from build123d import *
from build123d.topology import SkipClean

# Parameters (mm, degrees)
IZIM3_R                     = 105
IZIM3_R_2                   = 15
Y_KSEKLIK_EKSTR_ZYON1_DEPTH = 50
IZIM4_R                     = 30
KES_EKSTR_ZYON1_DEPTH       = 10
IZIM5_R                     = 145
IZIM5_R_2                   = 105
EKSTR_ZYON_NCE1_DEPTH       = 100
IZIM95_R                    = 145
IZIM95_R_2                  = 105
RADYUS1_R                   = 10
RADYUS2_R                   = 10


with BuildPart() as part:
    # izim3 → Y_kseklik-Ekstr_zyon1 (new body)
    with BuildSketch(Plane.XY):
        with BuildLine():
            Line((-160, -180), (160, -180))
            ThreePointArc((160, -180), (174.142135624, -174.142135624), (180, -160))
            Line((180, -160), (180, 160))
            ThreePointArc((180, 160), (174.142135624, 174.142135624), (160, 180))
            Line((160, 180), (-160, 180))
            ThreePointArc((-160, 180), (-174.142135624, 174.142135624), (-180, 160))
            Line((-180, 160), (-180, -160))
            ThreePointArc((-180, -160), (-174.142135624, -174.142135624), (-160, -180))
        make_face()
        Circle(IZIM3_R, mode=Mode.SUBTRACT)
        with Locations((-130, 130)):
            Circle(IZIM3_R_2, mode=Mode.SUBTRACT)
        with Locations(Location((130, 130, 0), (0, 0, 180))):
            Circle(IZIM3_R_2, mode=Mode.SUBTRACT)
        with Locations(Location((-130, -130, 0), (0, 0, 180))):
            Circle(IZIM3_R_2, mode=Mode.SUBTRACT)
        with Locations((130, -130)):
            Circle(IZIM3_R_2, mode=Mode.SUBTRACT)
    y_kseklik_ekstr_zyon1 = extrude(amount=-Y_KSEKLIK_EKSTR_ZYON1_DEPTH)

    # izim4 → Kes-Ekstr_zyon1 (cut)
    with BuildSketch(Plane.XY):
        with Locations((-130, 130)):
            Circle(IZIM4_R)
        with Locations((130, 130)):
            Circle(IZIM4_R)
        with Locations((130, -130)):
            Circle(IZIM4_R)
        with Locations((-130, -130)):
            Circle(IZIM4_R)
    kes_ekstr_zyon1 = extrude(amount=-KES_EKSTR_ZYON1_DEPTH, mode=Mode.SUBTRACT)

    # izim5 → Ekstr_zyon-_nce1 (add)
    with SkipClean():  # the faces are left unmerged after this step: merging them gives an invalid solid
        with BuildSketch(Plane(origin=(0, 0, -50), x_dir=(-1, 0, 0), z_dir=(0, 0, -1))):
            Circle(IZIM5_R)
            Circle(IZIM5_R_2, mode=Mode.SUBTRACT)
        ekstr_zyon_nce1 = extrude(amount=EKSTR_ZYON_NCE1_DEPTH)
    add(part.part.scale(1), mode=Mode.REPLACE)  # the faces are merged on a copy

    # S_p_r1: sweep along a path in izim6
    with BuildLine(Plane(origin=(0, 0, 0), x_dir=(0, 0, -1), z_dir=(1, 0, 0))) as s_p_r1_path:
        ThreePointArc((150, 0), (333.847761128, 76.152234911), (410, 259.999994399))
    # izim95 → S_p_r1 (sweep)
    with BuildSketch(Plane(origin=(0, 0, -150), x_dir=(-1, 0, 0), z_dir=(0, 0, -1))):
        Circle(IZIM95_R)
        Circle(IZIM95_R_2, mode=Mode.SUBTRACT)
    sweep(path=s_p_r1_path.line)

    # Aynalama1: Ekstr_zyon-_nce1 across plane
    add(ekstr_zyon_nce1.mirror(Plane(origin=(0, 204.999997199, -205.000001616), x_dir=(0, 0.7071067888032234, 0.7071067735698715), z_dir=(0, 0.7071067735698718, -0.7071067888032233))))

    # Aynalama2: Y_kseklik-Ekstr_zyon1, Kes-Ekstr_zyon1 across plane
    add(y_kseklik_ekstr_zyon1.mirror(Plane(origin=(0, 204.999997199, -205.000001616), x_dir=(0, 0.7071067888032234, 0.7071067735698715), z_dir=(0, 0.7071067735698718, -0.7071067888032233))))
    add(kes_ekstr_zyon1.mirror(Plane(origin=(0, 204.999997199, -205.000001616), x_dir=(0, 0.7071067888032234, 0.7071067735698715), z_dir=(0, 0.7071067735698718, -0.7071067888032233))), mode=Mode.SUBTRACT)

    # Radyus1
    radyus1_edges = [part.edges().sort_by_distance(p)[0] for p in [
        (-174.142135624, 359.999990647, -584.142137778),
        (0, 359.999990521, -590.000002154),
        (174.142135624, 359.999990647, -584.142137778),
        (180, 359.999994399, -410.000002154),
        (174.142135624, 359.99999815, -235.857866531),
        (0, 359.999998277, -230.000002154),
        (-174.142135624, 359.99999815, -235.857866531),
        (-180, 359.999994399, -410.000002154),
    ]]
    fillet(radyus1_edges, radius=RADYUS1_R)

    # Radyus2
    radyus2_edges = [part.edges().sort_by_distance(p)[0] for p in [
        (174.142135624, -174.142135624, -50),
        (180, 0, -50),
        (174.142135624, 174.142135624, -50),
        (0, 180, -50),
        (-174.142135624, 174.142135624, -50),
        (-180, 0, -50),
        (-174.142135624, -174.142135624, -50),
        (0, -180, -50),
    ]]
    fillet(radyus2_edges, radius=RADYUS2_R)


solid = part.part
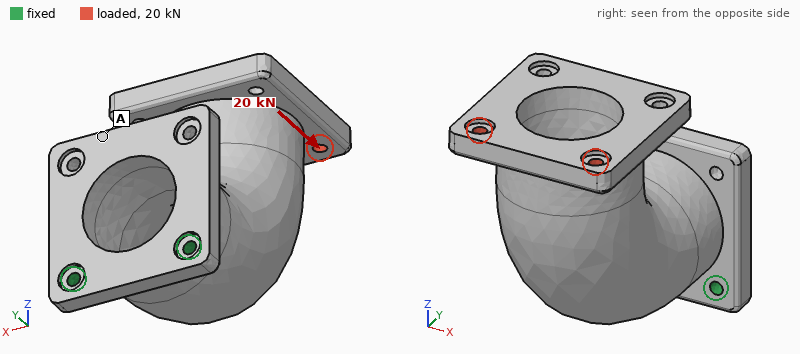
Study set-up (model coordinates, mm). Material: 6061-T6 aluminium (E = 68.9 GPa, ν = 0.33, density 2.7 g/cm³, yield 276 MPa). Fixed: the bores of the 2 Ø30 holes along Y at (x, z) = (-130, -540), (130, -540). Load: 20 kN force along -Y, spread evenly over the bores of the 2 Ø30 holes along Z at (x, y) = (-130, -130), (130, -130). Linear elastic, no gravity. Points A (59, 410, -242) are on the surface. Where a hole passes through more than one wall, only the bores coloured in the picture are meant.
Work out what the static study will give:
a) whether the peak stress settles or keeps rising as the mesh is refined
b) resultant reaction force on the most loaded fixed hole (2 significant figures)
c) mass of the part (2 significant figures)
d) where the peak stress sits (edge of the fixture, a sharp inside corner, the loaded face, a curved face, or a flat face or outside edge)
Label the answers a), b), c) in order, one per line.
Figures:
a) keeps rising
b) 10 kN
c) 76 kg
d) edge of the fixture
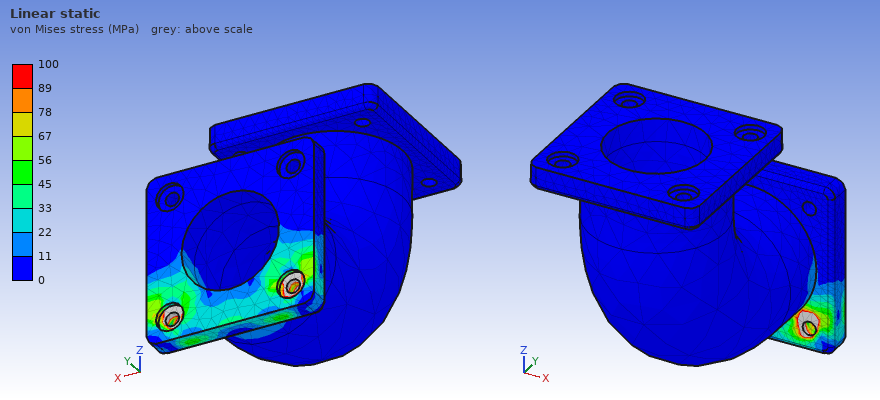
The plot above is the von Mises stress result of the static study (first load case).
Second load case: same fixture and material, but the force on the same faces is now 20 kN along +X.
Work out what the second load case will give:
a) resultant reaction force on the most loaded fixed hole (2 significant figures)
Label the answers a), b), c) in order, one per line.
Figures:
a) 57 kN
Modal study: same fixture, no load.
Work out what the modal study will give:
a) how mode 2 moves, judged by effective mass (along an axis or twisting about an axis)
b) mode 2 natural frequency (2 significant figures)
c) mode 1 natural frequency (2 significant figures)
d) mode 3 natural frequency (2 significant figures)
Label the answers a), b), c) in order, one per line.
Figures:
a) along X
b) 220 Hz
c) 68 Hz
d) 540 Hz
